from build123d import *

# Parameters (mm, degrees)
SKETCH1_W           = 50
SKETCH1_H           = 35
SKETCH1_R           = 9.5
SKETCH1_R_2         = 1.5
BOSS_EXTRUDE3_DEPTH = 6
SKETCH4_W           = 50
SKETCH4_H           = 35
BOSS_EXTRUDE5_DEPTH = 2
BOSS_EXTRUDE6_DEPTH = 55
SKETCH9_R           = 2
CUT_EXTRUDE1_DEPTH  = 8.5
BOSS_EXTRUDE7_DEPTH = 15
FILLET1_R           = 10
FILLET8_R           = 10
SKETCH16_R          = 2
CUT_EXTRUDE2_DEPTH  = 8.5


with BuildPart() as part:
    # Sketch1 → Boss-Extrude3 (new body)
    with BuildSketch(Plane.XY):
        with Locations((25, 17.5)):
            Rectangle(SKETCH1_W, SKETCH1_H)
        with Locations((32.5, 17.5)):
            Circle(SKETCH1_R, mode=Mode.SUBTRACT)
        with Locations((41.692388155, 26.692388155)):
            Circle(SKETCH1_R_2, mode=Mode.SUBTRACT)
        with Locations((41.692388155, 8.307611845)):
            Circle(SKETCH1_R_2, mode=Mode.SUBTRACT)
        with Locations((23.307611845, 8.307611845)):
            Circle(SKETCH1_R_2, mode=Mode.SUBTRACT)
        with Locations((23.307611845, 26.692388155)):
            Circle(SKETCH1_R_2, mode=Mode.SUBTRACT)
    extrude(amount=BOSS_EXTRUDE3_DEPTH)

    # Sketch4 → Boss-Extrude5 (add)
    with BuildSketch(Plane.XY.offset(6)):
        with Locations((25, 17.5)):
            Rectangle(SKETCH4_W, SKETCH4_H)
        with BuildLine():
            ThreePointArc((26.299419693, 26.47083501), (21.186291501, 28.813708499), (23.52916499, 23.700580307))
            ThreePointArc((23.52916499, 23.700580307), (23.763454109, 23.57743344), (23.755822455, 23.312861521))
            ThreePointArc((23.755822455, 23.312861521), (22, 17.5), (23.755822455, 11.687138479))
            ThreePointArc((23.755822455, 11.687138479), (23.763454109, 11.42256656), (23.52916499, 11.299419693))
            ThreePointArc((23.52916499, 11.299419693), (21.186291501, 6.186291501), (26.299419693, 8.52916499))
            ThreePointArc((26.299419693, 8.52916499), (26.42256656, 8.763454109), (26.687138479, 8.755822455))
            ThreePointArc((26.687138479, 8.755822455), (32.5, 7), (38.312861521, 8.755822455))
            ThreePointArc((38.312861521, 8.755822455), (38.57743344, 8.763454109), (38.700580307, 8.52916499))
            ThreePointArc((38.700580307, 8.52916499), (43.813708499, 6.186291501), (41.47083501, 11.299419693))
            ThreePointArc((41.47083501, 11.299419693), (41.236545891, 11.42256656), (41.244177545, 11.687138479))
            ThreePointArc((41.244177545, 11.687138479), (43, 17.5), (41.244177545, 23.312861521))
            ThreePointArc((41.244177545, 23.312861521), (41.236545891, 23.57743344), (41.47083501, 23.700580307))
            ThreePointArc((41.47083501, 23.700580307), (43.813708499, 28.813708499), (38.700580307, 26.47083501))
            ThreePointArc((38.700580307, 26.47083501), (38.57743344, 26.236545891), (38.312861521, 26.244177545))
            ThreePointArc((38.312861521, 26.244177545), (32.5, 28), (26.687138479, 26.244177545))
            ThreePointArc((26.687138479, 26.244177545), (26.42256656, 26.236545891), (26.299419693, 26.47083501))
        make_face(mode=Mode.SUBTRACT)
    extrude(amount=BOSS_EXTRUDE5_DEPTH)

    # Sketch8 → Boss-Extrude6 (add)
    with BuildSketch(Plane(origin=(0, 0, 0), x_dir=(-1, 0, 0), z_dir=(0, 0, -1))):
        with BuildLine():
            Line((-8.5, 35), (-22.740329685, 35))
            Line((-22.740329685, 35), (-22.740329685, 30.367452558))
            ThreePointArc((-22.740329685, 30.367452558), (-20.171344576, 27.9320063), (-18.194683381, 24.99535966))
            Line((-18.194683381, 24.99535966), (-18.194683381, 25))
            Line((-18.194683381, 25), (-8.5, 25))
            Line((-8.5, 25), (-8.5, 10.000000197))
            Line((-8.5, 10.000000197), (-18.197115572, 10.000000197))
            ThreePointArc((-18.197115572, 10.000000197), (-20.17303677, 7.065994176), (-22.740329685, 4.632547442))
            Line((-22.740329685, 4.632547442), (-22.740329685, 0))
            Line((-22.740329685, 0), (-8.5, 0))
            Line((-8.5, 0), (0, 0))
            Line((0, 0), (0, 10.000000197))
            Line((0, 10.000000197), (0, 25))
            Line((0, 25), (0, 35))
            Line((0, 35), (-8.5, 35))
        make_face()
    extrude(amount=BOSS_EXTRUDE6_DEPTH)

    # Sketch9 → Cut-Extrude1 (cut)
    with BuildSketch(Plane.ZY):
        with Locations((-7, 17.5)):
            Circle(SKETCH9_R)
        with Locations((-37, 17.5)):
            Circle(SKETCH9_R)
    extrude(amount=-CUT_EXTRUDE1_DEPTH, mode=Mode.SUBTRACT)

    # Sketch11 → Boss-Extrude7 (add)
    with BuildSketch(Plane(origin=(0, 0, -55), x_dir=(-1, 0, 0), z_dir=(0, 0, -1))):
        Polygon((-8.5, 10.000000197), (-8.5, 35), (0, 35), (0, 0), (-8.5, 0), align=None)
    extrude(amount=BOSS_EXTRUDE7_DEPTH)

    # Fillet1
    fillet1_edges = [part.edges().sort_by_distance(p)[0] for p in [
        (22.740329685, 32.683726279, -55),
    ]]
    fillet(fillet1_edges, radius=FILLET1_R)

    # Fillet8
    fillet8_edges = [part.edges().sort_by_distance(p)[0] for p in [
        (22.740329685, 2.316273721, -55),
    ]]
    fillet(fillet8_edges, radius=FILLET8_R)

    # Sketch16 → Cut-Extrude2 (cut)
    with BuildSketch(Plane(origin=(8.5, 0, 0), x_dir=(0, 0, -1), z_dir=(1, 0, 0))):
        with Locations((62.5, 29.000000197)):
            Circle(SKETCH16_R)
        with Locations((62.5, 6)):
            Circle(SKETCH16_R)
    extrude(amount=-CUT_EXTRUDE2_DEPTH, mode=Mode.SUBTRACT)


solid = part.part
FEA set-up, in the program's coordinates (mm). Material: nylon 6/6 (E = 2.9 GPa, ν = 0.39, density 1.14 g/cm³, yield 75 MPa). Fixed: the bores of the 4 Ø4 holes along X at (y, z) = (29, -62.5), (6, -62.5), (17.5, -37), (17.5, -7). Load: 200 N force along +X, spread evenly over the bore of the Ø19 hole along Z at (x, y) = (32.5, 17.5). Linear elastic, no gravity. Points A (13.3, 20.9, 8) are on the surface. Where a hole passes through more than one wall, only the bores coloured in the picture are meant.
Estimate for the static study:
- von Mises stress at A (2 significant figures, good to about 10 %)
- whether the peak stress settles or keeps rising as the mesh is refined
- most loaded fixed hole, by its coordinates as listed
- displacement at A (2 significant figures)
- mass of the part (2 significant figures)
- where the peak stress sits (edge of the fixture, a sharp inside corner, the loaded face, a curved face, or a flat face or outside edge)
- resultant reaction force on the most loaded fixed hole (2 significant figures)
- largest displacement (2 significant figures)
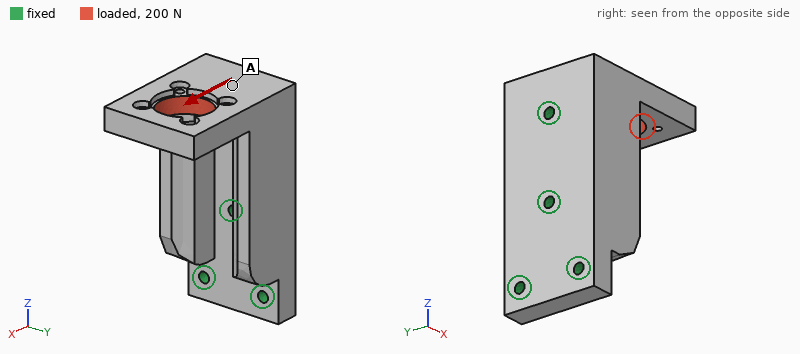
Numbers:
0.60 MPa
keeps rising
(17.5, -7)
23 µm
52 g
edge of the fixture
230 N
46 µm
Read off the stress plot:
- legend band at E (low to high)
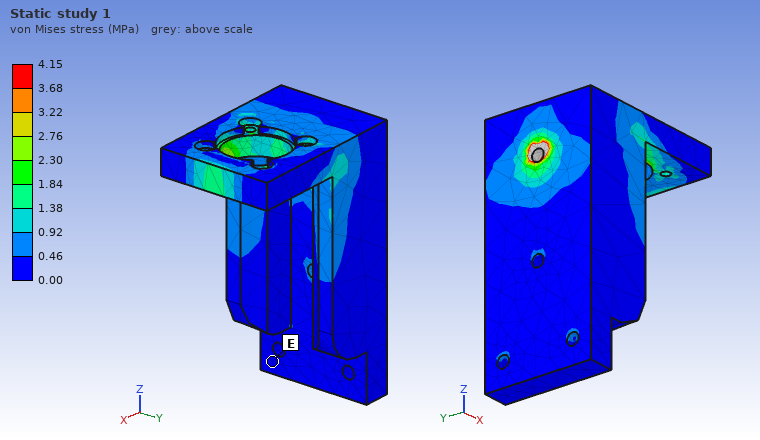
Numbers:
0.00 to 0.46 MPa
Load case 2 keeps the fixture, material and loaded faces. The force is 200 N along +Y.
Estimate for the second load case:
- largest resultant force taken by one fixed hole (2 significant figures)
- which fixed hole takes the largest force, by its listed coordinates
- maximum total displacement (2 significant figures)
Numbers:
230 N
(17.5, -7)
0.41 mm
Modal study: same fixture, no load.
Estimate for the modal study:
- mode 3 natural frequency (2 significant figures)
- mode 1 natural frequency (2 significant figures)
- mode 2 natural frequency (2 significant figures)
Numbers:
2800 Hz
1300 Hz
1300 Hz
